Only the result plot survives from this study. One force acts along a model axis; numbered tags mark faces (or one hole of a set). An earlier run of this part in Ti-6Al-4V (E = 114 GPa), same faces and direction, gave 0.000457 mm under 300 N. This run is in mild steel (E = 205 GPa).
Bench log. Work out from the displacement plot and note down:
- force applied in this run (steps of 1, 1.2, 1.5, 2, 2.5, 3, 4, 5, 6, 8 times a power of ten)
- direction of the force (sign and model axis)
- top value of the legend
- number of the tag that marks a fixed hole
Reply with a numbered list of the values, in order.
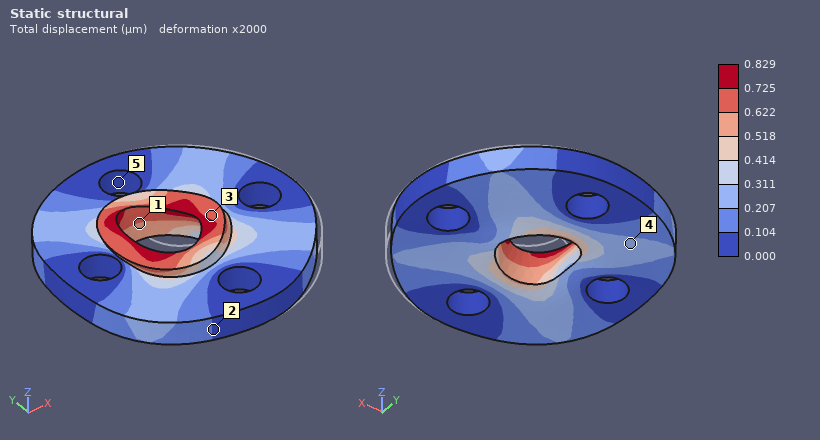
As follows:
1. 1 kN
2. -X
3. 0.829 µm
4. 5
